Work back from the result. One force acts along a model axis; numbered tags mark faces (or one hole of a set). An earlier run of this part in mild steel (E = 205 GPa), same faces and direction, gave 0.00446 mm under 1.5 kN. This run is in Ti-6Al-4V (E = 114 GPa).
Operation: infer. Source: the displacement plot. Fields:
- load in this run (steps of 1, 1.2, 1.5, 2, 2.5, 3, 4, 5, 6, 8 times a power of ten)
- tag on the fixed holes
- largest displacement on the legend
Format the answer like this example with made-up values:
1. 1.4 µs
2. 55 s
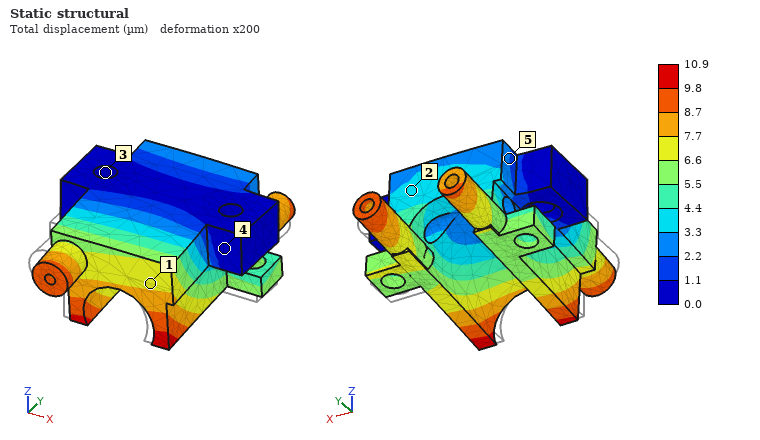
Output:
1. 2 kN
2. 3
3. 10.9 µm
